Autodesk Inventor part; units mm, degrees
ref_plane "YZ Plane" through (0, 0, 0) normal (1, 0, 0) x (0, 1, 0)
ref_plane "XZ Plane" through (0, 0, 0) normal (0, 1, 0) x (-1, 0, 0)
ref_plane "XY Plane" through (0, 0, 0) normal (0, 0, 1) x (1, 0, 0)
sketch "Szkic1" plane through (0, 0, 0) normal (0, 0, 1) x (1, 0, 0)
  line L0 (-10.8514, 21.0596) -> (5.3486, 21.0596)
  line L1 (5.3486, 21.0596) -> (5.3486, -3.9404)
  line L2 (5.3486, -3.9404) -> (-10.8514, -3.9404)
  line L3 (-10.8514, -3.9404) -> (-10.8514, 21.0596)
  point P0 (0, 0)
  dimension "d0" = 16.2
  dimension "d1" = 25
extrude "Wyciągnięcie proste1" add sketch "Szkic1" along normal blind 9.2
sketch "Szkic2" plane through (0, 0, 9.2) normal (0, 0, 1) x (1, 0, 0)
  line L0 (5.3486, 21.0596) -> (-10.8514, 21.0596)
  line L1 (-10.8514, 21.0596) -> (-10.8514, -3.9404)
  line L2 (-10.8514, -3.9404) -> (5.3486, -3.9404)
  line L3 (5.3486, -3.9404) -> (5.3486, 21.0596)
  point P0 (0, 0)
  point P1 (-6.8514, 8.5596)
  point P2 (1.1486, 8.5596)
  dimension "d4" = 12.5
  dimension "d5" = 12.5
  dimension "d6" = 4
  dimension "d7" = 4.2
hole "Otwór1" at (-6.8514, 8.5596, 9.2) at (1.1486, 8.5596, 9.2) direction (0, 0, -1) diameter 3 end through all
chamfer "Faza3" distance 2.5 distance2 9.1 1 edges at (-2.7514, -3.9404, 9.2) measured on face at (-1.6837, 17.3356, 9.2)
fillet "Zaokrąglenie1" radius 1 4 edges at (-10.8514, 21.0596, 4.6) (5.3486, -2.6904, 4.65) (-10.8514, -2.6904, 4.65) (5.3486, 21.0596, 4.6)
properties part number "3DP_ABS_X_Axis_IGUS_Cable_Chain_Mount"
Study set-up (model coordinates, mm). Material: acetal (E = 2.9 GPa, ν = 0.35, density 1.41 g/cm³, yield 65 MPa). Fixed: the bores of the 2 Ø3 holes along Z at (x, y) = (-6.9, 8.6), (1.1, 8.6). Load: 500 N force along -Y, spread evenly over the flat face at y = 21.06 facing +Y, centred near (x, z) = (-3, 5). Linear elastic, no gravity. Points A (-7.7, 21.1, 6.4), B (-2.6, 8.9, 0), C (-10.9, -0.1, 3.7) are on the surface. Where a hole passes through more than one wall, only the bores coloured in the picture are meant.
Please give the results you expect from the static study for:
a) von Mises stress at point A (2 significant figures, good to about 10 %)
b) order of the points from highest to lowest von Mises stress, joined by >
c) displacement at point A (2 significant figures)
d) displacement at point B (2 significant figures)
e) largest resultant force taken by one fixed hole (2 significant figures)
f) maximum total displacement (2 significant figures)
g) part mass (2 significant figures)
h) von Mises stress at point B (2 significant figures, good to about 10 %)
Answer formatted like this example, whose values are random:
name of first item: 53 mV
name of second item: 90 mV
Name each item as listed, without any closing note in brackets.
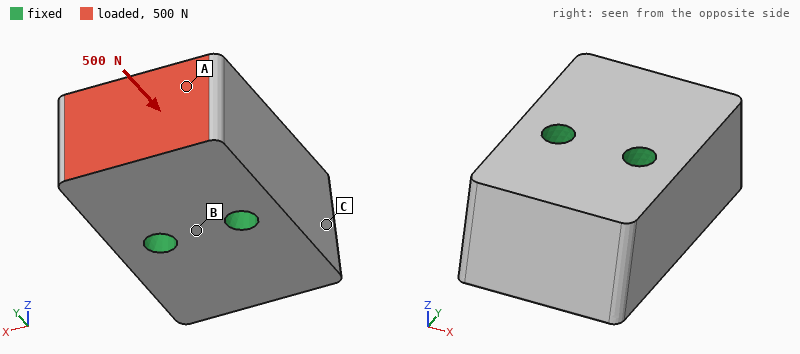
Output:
von Mises stress at point A: 3.1 MPa
order of the points from highest to lowest von Mises stress, joined by >: A > B > C
displacement at point A: 14 µm
displacement at point B: 2.6 µm
largest resultant force taken by one fixed hole: 260 N
maximum total displacement: 16 µm
part mass: 4.8 g
von Mises stress at point B: 1.4 MPa
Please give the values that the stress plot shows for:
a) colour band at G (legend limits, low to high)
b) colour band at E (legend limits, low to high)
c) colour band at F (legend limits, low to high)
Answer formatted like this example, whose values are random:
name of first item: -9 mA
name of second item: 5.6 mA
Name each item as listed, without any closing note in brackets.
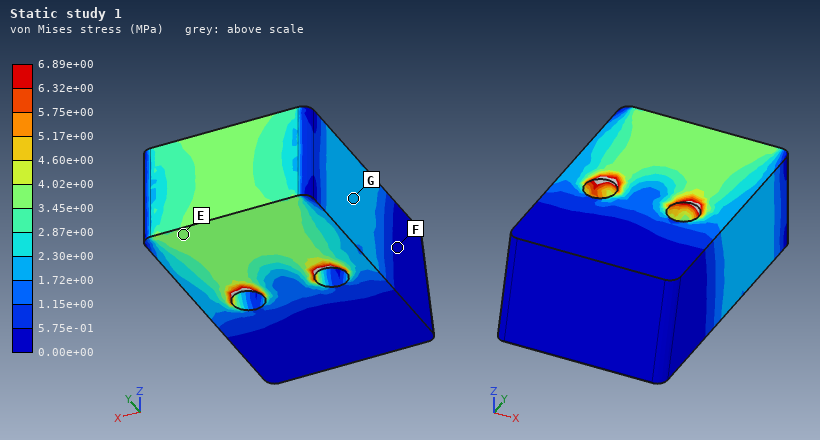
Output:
colour band at G: 1.72e+00 to 2.30e+00 MPa
colour band at E: 3.45e+00 to 4.02e+00 MPa
colour band at F: 0.00e+00 to 5.75e-01 MPa
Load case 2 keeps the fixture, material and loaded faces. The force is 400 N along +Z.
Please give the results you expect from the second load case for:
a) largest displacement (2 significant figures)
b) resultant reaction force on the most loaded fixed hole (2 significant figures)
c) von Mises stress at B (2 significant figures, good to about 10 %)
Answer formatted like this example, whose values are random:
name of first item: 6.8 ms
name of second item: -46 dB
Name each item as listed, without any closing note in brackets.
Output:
largest displacement: 0.13 mm
resultant reaction force on the most loaded fixed hole: 200 N
von Mises stress at B: 8.8 MPa
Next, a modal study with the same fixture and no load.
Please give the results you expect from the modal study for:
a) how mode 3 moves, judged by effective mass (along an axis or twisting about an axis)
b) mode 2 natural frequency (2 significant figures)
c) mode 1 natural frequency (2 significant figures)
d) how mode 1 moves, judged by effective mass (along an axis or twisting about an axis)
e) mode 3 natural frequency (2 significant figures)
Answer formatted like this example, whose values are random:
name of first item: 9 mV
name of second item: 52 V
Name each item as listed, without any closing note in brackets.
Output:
how mode 3 moves, judged by effective mass: along Z
mode 2 natural frequency: 12 kHz
mode 1 natural frequency: 11 kHz
how mode 1 moves, judged by effective mass: along Z
mode 3 natural frequency: 13 kHz
